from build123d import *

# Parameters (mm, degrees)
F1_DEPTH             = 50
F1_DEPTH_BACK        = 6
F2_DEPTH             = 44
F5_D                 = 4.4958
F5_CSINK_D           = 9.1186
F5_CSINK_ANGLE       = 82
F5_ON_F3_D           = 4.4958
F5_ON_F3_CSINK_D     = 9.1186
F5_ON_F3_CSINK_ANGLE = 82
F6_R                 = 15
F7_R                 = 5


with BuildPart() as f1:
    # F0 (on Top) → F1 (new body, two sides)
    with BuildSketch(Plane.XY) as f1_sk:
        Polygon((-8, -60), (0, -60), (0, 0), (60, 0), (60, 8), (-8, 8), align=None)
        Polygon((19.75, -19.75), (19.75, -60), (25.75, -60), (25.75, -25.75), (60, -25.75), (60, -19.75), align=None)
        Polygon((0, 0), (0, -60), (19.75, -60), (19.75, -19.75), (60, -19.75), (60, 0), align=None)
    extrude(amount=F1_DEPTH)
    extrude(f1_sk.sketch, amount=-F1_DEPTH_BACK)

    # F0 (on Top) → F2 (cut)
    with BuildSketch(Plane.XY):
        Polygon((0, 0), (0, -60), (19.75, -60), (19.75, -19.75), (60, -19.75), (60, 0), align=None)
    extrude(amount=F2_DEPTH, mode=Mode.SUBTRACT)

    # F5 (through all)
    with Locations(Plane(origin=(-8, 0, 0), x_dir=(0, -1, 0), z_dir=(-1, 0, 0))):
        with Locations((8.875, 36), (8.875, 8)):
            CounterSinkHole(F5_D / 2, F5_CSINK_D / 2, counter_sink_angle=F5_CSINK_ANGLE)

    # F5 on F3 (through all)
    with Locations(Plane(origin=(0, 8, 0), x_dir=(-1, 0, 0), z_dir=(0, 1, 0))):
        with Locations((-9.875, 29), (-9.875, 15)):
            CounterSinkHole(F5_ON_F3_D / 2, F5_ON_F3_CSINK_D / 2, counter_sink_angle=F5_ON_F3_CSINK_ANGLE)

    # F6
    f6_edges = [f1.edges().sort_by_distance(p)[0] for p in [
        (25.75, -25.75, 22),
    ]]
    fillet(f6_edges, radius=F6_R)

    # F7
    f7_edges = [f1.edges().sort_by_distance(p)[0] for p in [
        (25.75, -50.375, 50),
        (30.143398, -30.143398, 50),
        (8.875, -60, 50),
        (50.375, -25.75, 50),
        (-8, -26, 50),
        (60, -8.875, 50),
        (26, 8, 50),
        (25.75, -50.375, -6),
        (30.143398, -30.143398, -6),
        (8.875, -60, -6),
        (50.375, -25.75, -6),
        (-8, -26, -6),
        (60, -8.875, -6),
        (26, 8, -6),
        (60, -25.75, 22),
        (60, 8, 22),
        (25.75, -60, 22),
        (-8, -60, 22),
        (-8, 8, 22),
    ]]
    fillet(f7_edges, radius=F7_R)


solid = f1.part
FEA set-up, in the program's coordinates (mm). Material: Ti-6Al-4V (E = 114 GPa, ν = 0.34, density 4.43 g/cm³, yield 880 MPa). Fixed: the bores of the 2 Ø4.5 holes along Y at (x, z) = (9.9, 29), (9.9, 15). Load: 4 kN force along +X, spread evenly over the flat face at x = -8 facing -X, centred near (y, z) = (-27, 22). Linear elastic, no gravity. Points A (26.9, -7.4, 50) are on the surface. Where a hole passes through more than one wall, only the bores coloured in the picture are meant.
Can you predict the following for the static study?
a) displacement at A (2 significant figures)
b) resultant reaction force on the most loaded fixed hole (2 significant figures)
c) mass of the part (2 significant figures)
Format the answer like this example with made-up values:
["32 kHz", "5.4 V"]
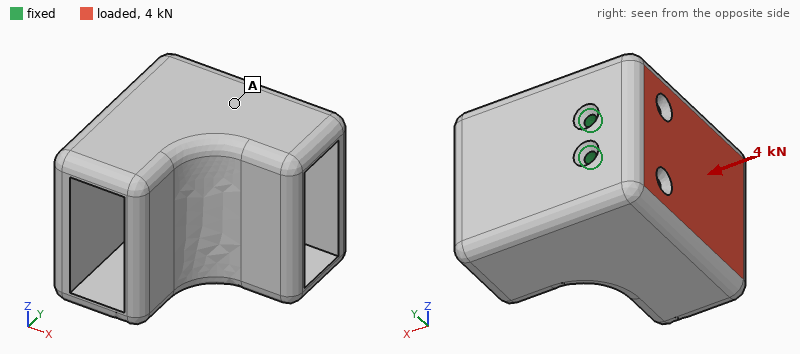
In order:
["0.11 mm", "2.0 kN", "460 g"]
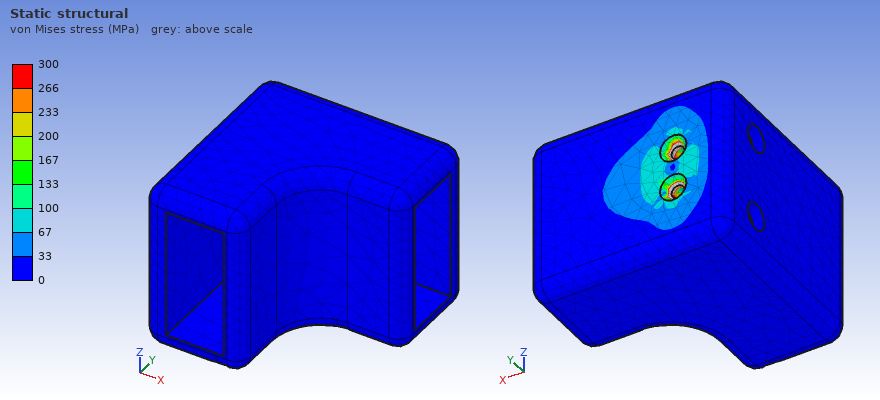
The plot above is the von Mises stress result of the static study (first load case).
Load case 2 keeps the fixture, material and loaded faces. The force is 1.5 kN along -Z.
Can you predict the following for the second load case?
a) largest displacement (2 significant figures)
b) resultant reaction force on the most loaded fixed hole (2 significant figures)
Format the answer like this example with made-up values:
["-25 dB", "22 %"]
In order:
["55 µm", "2.7 kN"]
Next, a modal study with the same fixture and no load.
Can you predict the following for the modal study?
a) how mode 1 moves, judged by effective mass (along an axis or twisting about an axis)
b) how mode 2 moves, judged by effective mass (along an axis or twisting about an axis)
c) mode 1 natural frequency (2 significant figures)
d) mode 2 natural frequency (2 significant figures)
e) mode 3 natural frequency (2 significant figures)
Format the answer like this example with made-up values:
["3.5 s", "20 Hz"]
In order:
["along X", "along Z", "960 Hz", "1600 Hz", "3100 Hz"]
